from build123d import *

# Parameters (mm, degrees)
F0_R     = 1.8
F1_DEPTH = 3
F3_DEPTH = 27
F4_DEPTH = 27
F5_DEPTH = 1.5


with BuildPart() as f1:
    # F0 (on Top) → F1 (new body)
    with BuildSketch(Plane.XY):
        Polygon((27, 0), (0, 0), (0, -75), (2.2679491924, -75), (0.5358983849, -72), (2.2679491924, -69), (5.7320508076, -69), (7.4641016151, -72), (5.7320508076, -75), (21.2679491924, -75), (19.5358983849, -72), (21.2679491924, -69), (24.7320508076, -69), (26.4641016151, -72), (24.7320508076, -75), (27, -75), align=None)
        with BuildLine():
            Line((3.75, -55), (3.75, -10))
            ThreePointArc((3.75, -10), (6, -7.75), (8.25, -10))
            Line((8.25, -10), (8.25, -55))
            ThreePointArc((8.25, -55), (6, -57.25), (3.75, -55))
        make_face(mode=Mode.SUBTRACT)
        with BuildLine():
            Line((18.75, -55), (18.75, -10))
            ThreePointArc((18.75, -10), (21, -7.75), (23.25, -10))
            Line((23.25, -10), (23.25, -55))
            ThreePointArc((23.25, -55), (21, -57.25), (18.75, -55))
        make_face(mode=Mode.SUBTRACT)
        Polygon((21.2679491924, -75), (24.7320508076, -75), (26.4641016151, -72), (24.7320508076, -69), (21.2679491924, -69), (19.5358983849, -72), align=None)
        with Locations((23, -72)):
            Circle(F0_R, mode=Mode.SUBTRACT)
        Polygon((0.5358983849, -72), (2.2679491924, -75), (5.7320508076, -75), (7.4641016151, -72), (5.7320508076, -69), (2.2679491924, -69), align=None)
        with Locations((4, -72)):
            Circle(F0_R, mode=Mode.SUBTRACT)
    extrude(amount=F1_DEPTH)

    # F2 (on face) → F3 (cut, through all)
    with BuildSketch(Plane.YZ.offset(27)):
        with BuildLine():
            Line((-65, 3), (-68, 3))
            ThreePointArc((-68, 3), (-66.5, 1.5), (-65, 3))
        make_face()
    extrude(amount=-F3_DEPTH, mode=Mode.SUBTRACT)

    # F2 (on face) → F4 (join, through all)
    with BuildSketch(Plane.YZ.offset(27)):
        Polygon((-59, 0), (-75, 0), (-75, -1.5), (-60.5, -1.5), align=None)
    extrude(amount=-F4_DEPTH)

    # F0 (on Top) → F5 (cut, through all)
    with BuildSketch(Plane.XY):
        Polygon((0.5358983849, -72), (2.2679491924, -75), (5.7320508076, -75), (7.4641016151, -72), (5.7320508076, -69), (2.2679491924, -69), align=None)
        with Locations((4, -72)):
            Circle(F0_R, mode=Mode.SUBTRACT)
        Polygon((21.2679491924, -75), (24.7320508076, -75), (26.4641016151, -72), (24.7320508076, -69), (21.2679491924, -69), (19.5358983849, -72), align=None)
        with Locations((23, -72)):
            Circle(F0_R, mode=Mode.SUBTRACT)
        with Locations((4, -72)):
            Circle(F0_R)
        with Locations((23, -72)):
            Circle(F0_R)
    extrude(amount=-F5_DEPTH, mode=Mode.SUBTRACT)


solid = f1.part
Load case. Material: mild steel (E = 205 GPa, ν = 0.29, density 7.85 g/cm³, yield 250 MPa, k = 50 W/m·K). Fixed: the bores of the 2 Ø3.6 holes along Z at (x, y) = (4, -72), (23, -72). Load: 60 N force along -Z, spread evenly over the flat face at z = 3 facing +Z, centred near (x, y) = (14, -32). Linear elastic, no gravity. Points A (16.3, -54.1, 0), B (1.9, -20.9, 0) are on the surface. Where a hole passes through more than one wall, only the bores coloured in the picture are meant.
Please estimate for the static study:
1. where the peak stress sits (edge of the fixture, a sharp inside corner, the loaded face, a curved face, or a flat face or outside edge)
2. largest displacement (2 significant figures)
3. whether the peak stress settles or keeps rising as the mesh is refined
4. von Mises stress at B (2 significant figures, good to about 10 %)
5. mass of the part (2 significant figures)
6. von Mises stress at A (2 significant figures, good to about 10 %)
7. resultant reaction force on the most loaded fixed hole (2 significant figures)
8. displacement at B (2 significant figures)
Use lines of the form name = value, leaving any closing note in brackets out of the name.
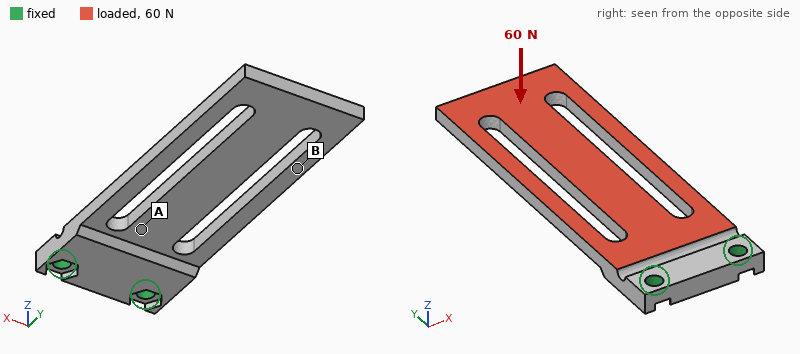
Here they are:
where the peak stress sits = edge of the fixture
largest displacement = 0.26 mm
whether the peak stress settles or keeps rising as the mesh is refined = keeps rising
von Mises stress at B = 8.5 MPa
mass of the part = 40 g
von Mises stress at A = 49 MPa
resultant reaction force on the most loaded fixed hole = 33 N
displacement at B = 0.15 mm
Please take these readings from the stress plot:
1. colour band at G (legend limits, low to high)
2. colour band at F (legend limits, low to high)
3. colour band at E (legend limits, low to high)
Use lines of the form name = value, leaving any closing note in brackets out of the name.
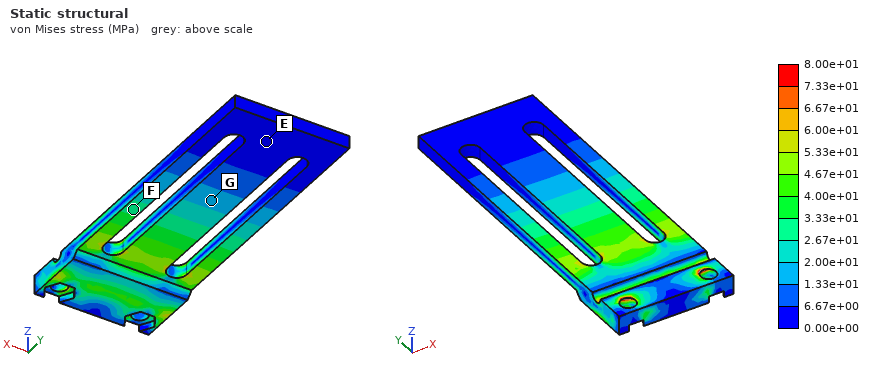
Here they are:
colour band at G = 1.33e+01 to 2.00e+01 MPa
colour band at F = 2.67e+01 to 3.33e+01 MPa
colour band at E = 0.00e+00 to 6.67e+00 MPa
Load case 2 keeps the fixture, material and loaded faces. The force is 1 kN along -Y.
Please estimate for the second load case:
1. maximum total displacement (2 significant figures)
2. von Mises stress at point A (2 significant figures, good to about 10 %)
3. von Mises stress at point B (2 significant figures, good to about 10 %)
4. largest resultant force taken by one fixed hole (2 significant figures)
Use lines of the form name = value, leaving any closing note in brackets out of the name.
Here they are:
maximum total displacement = 0.28 mm
von Mises stress at point A = 29 MPa
von Mises stress at point B = 13 MPa
largest resultant force taken by one fixed hole = 510 N
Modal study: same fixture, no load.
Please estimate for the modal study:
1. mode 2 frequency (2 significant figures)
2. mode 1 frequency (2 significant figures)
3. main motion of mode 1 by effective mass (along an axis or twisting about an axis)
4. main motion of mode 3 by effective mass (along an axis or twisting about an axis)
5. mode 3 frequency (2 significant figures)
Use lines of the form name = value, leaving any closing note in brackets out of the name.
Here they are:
mode 2 frequency = 2400 Hz
mode 1 frequency = 530 Hz
main motion of mode 1 by effective mass = along Z
main motion of mode 3 by effective mass = along X
mode 3 frequency = 2500 Hz
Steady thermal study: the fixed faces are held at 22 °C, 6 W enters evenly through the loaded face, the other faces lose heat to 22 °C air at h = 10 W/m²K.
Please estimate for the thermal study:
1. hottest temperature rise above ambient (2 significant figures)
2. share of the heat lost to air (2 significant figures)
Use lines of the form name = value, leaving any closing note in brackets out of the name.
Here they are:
hottest temperature rise above ambient = 60 K
share of the heat lost to air = 17 %
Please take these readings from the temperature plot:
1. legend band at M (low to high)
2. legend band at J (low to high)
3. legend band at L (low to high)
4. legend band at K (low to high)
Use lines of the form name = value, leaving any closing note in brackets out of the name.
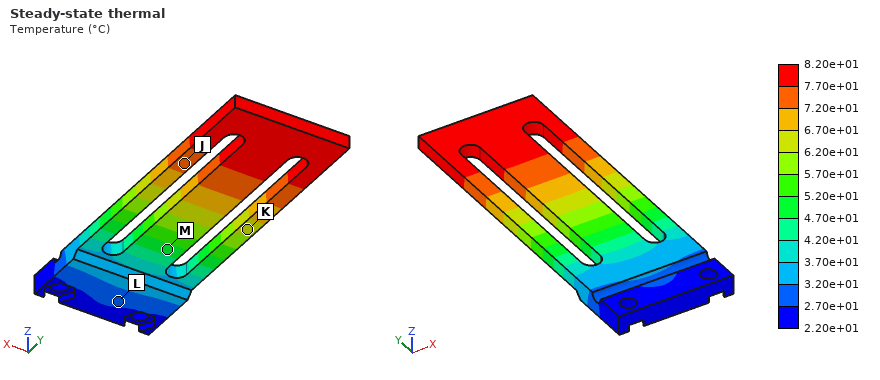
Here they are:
legend band at M = 4.70e+01 to 5.20e+01 °C
legend band at J = 7.20e+01 to 7.70e+01 °C
legend band at L = 2.70e+01 to 3.20e+01 °C
legend band at K = 6.20e+01 to 6.70e+01 °C
